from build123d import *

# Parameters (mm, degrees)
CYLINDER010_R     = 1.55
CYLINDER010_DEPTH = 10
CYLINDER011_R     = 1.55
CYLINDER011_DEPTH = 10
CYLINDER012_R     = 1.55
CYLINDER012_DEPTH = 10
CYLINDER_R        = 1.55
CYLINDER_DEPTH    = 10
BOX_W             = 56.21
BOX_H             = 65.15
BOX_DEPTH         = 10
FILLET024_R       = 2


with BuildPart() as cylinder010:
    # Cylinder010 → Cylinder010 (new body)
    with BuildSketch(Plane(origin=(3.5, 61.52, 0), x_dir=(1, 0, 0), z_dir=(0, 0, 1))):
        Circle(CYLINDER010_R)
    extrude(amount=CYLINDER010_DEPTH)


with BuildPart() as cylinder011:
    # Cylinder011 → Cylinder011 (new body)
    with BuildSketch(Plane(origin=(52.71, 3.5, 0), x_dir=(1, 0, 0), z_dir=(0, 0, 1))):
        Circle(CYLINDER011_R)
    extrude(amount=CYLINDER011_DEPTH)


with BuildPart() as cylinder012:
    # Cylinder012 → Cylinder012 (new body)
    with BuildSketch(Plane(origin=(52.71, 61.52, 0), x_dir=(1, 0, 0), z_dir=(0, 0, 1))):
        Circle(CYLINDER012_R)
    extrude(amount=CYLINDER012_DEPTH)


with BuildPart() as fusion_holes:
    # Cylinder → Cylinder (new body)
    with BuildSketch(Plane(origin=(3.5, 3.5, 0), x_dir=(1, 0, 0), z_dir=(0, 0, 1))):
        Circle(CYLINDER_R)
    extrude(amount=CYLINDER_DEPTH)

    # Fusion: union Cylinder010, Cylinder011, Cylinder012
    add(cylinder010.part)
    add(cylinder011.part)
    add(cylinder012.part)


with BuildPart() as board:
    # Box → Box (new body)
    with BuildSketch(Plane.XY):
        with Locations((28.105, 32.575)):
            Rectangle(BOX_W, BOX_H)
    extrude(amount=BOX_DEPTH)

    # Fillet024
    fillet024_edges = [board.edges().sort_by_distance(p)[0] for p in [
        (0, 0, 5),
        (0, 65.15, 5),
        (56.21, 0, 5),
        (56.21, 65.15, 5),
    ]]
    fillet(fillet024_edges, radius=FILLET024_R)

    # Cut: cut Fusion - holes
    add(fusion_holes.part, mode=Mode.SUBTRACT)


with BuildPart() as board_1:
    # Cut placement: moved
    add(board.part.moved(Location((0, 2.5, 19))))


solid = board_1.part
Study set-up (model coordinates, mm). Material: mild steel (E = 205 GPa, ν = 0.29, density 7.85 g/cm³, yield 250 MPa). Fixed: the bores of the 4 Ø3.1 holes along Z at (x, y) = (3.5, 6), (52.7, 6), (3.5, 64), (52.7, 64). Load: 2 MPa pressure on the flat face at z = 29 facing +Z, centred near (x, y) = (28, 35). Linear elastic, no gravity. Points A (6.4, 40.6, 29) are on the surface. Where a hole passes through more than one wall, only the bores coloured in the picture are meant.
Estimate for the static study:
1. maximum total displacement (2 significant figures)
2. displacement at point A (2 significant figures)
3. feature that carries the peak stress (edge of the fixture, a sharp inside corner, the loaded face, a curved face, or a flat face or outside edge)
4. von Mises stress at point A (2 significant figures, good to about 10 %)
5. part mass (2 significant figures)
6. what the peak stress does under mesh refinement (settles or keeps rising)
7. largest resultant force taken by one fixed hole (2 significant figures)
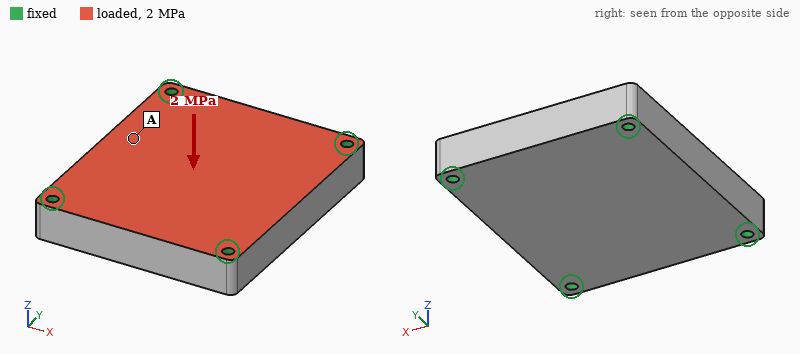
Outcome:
11 µm
8.3 µm
edge of the fixture
23 MPa
280 g
keeps rising
1.8 kN
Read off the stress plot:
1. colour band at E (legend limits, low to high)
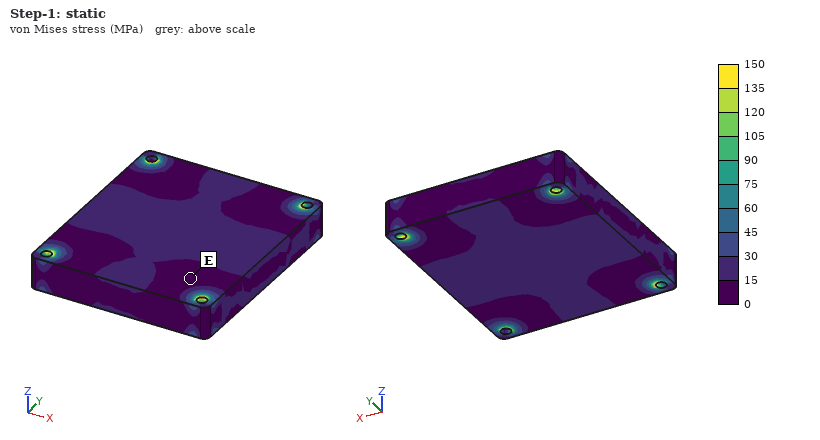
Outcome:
0 to 15 MPa
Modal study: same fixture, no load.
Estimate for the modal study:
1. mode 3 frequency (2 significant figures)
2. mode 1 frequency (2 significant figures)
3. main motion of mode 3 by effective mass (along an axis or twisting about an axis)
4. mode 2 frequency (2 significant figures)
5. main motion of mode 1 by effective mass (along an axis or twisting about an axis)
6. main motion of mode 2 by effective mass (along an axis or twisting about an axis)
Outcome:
17 kHz
9000 Hz
twisting about X
14 kHz
along Z
twisting about Y
